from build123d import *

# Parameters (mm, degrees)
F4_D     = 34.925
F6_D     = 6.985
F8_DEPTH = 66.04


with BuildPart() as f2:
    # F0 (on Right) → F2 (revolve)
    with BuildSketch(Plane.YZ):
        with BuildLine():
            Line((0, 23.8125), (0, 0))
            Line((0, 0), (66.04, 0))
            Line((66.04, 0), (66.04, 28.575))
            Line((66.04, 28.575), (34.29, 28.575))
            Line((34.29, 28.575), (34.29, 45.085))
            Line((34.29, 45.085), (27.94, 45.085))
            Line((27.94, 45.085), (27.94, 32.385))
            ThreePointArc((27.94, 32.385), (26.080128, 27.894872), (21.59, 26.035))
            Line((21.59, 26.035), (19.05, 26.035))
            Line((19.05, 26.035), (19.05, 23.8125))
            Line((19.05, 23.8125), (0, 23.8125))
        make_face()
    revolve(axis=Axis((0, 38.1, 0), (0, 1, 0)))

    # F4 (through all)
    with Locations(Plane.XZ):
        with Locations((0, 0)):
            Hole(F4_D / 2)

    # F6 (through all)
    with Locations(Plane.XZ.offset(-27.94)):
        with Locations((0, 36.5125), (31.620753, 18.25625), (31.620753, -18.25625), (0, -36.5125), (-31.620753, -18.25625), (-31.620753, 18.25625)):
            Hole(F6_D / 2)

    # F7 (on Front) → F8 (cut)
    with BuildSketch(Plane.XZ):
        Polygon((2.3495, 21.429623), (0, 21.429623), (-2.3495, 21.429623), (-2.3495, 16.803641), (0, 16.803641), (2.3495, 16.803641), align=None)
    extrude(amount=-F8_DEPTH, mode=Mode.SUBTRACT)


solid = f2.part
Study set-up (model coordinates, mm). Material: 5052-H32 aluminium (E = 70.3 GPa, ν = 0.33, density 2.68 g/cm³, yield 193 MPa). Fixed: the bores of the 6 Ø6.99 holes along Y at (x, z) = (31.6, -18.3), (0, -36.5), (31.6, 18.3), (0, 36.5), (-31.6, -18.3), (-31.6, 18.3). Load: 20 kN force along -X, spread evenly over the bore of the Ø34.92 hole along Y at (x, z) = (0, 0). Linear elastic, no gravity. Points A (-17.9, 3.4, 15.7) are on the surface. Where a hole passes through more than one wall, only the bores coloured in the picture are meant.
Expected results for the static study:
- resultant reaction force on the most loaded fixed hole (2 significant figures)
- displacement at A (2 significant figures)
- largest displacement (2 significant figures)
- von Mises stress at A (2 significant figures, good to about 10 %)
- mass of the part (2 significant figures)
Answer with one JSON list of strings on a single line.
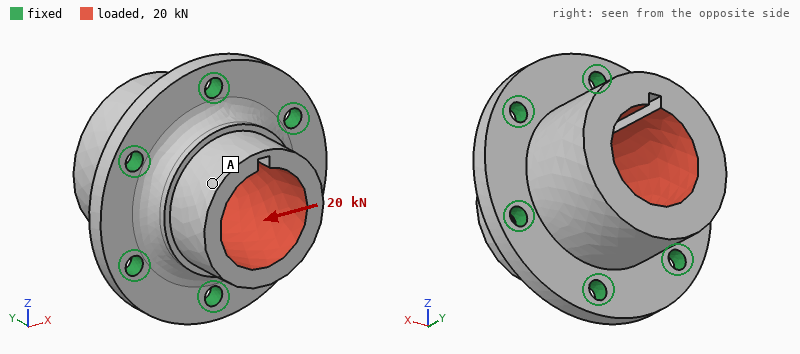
["4.1 kN", "14 µm", "17 µm", "8.3 MPa", "300 g"]
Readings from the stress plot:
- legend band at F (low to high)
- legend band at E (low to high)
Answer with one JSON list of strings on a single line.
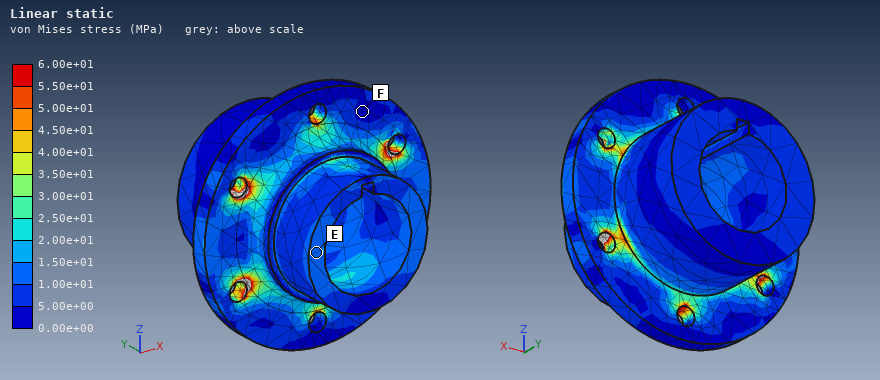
["0.00e+00 to 5.00e+00 MPa", "1.00e+01 to 1.50e+01 MPa"]
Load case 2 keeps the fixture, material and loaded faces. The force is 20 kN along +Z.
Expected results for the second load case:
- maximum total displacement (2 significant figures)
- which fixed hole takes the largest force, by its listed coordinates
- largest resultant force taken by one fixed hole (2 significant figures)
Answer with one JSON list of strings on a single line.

["18 µm", "(0, -36.5)", "4.6 kN"]
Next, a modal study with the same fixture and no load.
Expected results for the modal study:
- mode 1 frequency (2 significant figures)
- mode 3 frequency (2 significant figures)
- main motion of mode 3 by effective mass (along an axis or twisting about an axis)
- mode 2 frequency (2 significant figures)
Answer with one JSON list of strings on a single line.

["10000 Hz", "12 kHz", "along Y", "10 kHz"]
